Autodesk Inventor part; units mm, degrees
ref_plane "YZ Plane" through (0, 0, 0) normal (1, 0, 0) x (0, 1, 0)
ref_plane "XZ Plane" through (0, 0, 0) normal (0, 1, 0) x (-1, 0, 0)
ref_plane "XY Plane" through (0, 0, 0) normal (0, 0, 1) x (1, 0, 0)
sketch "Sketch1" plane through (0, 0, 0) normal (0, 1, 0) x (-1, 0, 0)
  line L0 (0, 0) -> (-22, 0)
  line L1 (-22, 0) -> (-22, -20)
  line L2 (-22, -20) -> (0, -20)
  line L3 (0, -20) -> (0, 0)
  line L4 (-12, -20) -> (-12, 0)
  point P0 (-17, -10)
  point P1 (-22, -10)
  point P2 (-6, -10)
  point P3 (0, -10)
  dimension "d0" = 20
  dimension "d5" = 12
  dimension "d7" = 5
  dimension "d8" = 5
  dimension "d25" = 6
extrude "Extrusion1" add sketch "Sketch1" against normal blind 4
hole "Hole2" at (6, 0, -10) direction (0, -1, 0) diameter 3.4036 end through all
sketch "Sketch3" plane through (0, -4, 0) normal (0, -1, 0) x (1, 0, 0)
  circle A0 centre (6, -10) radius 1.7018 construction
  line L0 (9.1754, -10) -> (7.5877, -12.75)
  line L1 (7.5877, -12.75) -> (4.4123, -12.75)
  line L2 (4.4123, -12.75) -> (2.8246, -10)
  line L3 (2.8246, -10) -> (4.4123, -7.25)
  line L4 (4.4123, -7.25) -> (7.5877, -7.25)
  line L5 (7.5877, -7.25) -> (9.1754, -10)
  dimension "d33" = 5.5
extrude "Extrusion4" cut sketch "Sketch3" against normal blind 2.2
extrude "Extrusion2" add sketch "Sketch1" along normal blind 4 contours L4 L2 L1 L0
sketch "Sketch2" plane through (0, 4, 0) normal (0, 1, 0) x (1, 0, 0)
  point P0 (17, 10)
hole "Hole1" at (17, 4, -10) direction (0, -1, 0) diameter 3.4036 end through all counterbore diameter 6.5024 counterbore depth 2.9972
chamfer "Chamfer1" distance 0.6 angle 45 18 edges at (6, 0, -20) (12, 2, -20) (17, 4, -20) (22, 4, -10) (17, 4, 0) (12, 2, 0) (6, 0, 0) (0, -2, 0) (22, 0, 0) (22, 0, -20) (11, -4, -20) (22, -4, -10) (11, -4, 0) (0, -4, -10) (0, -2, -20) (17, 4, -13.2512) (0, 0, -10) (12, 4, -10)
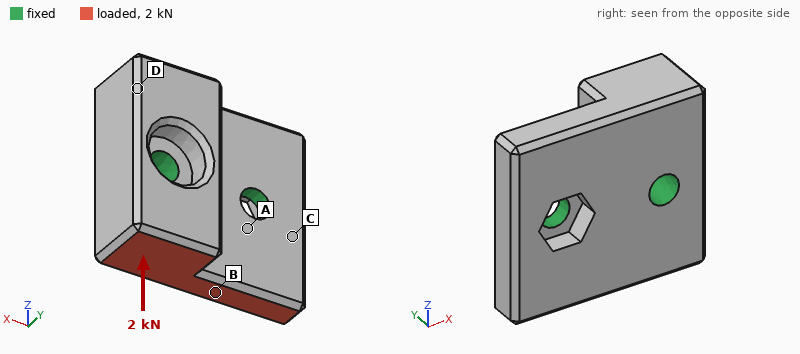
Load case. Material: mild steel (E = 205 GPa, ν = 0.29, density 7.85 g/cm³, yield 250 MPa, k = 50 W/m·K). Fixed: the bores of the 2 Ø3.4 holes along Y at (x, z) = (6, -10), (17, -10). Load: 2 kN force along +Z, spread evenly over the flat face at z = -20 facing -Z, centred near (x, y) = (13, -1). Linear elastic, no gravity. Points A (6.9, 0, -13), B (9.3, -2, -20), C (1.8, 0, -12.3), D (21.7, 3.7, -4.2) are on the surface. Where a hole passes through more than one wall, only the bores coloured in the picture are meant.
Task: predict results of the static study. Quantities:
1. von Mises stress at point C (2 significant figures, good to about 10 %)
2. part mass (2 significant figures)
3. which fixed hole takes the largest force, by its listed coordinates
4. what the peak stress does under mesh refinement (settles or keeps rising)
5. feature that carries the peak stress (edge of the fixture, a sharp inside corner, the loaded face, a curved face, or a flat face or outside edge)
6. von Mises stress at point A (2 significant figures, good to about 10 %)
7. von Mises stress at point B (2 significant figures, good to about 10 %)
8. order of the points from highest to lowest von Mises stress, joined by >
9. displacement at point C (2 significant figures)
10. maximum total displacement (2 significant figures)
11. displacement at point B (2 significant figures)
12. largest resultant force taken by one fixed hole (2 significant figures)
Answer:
10 MPa
18 g
(17, -10)
keeps rising
edge of the fixture
37 MPa
21 MPa
A > B > C > D
0.58 µm
2.0 µm
1.1 µm
1.3 kN
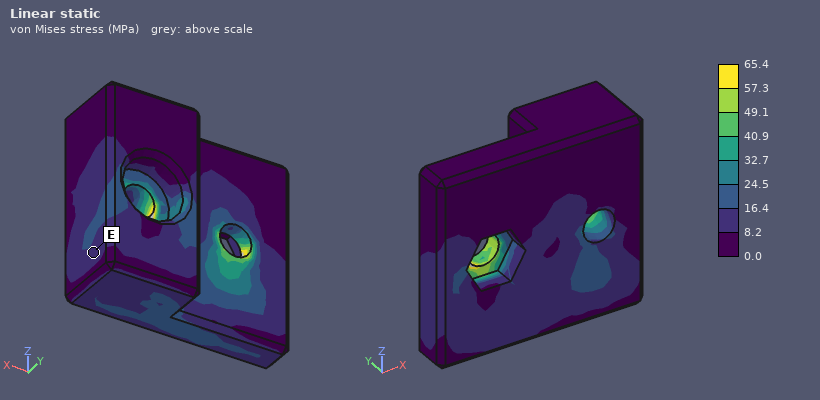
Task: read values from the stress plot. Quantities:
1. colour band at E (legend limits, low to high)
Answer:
8.2 to 16.4 MPa
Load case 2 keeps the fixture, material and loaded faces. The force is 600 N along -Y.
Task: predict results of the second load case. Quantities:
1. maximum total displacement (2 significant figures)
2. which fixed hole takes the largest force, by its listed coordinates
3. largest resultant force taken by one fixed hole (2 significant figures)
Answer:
8.4 µm
(17, -10)
440 N
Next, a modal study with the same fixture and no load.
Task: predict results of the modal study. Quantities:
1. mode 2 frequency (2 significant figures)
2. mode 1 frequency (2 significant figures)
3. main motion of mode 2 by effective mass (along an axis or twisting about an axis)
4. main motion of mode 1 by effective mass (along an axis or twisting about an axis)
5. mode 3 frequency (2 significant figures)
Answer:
32 kHz
23 kHz
along Y
twisting about X
35 kHz
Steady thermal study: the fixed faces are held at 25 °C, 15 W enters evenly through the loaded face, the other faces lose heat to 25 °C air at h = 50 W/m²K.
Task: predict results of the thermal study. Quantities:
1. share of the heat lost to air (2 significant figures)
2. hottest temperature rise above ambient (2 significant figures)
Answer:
3.8 %
29 K
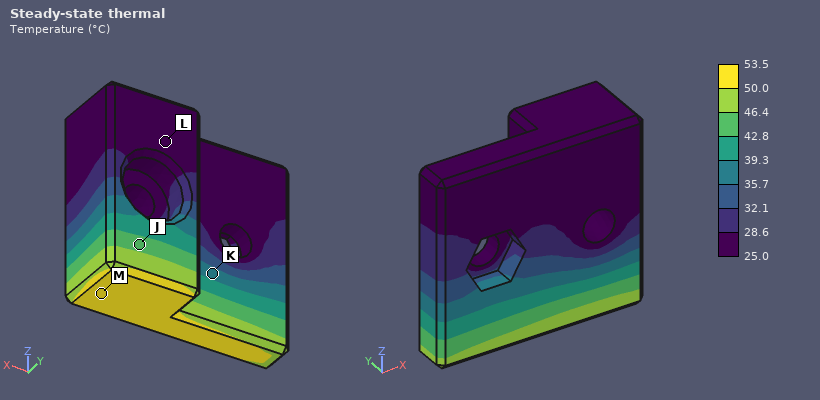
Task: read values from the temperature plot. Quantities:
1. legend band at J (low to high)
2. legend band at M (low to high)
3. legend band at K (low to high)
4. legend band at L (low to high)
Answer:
42.8 to 46.4 °C
50.0 to 53.5 °C
35.7 to 39.3 °C
25.0 to 28.6 °C
